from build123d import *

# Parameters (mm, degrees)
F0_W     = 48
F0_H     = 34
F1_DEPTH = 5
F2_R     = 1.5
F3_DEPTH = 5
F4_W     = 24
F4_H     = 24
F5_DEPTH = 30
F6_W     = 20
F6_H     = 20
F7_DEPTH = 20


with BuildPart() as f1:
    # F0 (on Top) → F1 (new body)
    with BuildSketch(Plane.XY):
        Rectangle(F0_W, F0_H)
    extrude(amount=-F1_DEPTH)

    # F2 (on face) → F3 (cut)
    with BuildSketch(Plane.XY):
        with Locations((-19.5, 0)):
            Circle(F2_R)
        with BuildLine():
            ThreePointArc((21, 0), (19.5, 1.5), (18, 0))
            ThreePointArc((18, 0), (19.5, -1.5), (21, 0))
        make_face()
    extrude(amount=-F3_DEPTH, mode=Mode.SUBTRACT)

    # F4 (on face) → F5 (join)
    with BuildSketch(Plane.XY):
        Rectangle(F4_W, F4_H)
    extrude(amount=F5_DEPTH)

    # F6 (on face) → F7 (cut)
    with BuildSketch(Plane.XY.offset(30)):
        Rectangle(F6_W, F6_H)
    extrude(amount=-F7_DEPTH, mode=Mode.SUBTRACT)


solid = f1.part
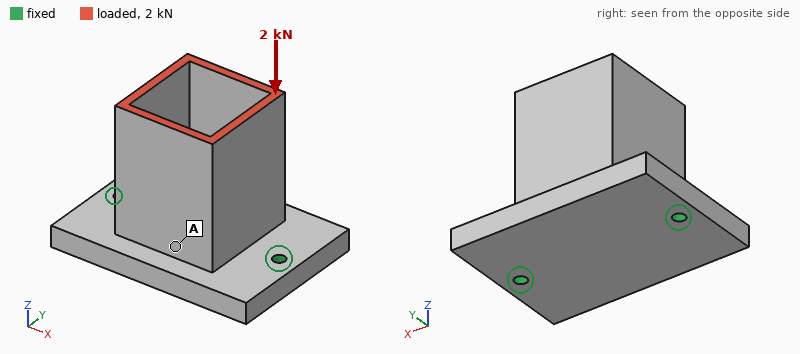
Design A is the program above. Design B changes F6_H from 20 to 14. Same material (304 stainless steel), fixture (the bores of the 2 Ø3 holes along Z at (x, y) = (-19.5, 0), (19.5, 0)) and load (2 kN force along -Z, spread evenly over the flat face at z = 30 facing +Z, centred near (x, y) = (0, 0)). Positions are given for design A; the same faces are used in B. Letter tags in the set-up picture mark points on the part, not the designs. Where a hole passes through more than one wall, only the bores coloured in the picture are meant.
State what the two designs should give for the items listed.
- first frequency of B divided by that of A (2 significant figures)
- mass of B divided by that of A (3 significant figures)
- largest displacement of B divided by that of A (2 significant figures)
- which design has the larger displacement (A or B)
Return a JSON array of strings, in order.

["0.84", "1.14", "0.91", "A"]
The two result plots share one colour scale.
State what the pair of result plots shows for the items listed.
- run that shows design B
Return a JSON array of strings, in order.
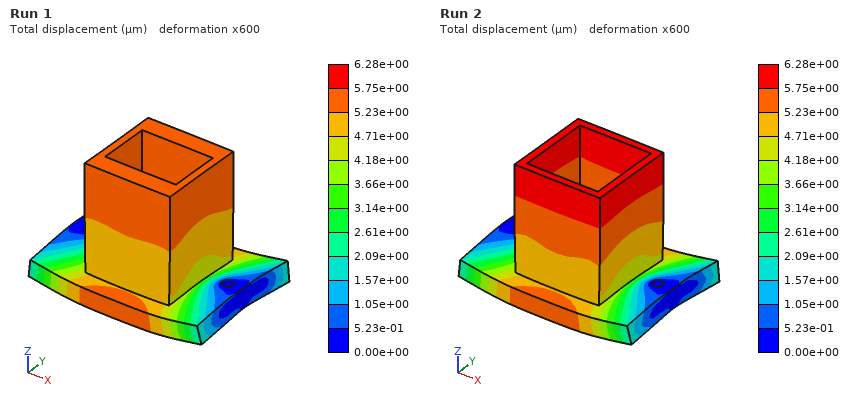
["Run 1"]
